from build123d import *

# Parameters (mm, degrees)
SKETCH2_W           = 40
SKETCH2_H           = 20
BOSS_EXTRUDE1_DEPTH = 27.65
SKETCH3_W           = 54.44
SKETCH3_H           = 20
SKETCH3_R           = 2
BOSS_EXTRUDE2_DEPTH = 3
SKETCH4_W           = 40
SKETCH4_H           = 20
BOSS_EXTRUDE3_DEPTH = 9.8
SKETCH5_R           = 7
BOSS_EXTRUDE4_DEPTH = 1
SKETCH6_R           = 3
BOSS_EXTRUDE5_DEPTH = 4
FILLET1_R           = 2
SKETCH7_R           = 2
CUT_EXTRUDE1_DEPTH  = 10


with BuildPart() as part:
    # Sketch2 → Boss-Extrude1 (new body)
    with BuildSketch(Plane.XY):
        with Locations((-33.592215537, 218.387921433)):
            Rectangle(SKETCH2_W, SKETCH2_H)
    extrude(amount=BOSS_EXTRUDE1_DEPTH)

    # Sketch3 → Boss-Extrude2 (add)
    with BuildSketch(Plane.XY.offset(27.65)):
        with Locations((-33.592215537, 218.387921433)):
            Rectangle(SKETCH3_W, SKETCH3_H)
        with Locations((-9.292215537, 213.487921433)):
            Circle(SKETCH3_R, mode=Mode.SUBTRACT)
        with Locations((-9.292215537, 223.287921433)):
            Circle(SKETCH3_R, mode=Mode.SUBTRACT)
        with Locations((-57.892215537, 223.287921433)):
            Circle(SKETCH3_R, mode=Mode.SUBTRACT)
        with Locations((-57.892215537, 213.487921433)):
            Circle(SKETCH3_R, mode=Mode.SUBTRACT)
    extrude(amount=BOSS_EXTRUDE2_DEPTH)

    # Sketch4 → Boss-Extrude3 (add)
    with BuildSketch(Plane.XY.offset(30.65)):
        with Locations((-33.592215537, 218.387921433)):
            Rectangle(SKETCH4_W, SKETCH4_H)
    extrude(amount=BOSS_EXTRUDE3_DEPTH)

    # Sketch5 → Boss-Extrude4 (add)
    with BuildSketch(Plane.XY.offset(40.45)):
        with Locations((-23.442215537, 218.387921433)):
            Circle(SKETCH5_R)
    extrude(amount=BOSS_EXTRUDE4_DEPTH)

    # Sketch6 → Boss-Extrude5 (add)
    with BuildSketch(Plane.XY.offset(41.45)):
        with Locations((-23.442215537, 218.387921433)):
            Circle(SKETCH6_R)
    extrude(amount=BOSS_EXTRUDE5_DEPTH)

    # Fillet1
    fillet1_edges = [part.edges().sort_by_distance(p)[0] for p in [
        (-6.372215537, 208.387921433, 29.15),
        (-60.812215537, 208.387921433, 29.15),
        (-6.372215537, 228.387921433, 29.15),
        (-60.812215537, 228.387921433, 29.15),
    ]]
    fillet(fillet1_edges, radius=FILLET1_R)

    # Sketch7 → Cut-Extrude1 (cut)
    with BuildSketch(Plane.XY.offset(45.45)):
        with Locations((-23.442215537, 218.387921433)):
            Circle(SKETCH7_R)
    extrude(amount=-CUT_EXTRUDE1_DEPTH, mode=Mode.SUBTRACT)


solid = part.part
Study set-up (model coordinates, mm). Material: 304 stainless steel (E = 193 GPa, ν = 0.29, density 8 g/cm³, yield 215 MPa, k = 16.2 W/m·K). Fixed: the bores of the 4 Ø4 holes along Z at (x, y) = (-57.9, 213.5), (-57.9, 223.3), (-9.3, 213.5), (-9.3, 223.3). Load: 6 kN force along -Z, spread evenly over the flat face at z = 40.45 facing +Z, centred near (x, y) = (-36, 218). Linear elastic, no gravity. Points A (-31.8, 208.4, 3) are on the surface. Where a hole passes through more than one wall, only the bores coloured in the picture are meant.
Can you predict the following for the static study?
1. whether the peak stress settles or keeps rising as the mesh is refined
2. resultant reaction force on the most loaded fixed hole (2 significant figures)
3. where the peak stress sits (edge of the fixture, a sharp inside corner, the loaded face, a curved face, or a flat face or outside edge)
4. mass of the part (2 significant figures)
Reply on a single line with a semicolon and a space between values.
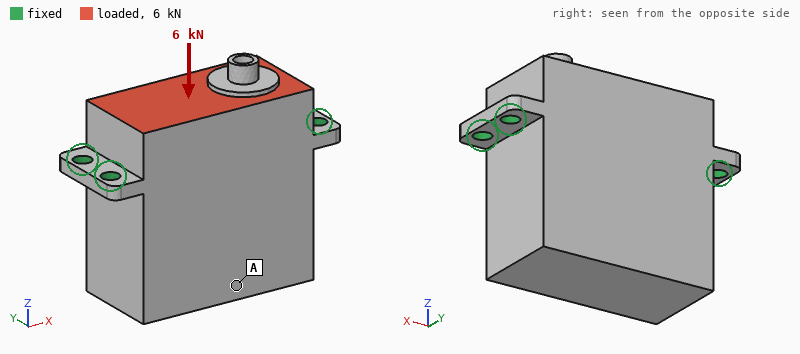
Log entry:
keeps rising; 1.7 kN; edge of the fixture; 270 g
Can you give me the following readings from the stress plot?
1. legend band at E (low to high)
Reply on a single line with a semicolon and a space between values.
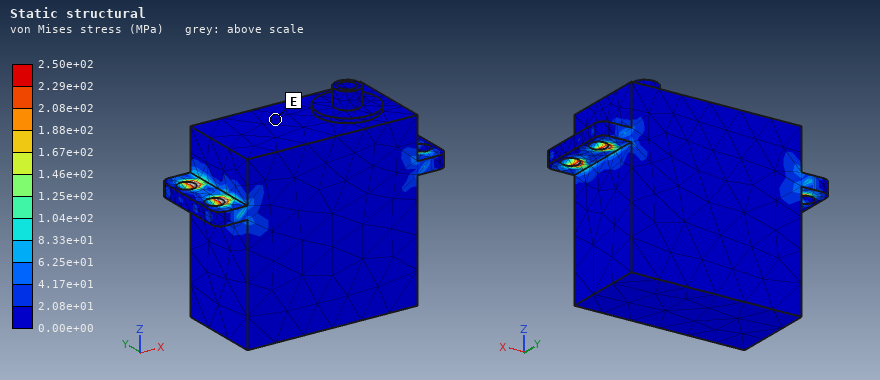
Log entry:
0.00e+00 to 2.08e+01 MPa
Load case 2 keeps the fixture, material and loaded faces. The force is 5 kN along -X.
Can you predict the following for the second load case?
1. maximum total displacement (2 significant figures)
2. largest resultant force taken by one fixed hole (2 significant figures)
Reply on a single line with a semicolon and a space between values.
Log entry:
5.2 µm; 1.5 kN
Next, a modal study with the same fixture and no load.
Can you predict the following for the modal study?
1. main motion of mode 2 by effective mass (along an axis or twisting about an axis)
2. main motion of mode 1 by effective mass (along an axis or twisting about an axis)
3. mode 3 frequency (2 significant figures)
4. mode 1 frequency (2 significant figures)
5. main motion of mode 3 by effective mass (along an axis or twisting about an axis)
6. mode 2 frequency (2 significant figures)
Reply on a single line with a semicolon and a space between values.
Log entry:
along Z; along Y; 10 kHz; 3500 Hz; along X; 9700 Hz
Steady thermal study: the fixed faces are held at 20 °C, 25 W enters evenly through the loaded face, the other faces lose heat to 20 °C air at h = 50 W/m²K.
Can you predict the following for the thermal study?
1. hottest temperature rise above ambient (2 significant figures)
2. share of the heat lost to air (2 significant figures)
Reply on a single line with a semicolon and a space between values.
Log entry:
66 K; 45 %
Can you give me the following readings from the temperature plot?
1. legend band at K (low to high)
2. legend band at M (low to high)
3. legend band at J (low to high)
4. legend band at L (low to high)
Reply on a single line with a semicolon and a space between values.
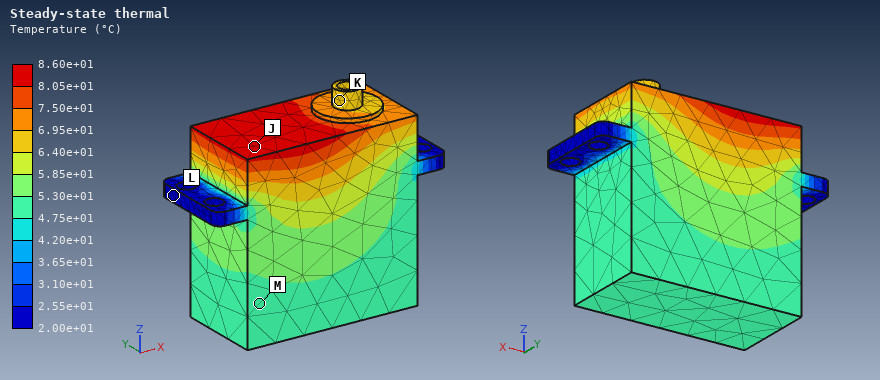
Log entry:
6.40e+01 to 6.95e+01 °C; 4.75e+01 to 5.30e+01 °C; 8.05e+01 to 8.60e+01 °C; 2.00e+01 to 2.55e+01 °C
